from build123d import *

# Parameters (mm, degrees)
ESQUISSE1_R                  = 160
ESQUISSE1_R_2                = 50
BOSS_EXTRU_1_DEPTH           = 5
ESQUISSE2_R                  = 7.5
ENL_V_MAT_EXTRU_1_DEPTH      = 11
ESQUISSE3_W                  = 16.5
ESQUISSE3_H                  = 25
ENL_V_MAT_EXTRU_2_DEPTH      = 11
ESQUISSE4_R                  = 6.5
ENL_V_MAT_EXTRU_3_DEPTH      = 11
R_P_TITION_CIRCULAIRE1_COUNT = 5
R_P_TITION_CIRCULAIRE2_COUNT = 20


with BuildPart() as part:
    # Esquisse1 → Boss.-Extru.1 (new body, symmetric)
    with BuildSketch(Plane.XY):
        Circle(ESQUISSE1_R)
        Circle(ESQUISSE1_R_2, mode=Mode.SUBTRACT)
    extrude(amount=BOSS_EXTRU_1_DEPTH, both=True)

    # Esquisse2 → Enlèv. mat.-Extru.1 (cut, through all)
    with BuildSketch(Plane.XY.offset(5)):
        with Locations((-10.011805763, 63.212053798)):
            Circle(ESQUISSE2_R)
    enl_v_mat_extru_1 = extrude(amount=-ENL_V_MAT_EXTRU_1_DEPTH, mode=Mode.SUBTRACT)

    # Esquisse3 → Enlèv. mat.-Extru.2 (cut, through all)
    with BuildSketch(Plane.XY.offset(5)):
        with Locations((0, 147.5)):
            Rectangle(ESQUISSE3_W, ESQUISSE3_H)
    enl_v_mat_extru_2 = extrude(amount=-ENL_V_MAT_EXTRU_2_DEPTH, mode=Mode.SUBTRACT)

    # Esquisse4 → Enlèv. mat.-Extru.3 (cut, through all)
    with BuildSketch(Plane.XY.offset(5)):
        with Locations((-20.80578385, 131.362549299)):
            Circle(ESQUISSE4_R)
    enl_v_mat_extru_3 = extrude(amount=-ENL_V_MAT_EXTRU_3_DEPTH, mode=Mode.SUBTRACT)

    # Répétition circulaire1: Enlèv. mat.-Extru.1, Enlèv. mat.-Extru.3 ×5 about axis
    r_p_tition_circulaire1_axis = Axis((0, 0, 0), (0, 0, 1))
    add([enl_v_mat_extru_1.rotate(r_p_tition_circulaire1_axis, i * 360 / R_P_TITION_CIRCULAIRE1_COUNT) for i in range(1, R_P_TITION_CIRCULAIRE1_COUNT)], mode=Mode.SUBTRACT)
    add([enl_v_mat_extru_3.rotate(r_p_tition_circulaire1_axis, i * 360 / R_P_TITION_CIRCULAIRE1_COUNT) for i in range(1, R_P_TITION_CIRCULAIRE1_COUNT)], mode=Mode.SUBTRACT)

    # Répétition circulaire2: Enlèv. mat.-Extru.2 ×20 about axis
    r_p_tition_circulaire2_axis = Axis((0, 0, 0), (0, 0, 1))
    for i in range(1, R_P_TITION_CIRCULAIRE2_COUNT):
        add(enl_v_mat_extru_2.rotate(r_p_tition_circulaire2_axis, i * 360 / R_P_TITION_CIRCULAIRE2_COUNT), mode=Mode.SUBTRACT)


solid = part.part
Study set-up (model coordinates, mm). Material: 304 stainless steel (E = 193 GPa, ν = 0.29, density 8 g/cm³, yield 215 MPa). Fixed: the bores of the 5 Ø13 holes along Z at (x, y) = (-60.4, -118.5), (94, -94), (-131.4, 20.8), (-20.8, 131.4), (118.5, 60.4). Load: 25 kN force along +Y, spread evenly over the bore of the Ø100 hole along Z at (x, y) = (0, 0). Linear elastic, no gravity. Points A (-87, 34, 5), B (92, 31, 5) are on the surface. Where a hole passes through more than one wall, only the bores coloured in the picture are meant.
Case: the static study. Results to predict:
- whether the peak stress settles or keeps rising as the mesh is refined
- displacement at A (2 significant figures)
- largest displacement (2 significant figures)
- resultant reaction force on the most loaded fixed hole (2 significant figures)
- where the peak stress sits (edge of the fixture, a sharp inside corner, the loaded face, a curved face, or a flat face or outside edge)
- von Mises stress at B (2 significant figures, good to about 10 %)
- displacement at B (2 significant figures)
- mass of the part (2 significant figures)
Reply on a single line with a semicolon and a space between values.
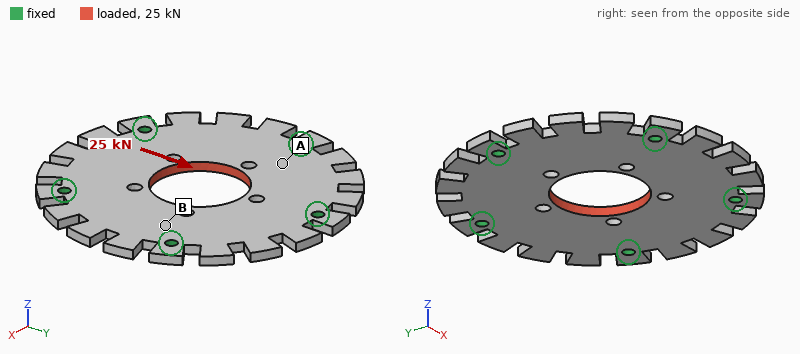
keeps rising; 3.2 µm; 7.1 µm; 6.8 kN; edge of the fixture; 8.1 MPa; 2.4 µm; 5.0 kg
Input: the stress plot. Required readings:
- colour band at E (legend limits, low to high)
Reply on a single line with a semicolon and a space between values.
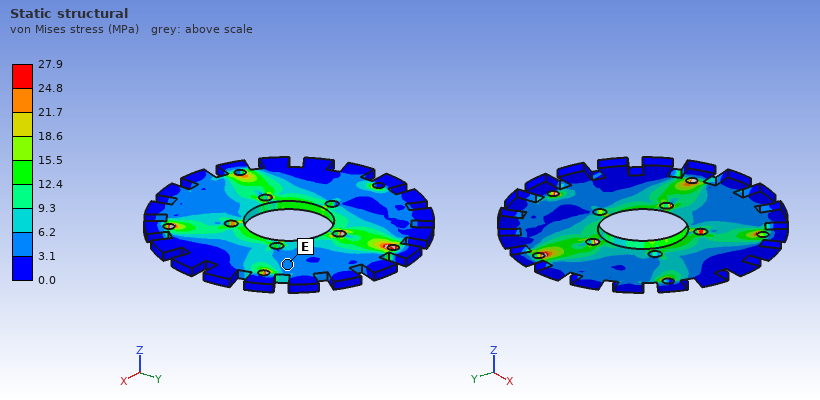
3.1 to 6.2 MPa
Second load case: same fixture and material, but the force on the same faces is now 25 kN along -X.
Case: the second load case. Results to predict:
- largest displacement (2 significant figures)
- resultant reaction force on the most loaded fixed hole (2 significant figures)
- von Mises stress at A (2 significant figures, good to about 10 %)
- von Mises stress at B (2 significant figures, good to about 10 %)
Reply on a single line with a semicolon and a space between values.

7.2 µm; 6.8 kN; 12 MPa; 11 MPa
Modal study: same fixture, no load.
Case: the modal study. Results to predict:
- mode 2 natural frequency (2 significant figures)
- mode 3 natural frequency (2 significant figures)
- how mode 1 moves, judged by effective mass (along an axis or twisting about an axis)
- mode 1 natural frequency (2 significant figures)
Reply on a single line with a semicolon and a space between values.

1400 Hz; 1400 Hz; along Z; 1200 Hz
